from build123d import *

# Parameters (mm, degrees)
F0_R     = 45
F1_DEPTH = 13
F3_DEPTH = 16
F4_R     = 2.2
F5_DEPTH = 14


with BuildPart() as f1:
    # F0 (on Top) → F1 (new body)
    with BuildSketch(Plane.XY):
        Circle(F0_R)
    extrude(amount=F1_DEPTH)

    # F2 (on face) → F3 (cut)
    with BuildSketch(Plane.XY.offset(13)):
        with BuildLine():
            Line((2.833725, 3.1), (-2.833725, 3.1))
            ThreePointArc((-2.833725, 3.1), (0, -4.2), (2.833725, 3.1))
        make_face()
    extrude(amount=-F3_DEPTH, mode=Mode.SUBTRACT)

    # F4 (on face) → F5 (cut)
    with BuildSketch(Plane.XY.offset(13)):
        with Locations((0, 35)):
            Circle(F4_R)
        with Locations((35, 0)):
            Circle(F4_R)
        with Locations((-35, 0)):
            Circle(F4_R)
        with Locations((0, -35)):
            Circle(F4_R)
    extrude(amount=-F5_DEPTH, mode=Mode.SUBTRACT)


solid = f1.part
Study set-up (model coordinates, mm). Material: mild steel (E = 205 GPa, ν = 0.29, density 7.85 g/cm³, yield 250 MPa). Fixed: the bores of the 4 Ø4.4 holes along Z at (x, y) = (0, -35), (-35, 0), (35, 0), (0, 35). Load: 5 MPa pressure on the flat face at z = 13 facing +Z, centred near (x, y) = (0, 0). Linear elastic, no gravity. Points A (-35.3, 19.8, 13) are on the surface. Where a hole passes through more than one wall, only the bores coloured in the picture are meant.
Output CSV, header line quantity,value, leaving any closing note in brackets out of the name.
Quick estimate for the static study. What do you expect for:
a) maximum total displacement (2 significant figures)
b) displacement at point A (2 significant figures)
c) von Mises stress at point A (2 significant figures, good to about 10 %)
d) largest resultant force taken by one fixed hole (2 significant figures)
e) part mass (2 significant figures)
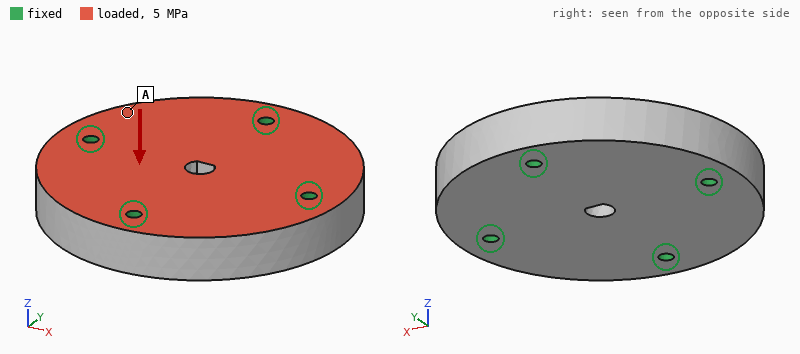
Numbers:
quantity,value
maximum total displacement,8.7 µm
displacement at point A,5.6 µm
von Mises stress at point A,15 MPa
largest resultant force taken by one fixed hole,7.8 kN
part mass,640 g
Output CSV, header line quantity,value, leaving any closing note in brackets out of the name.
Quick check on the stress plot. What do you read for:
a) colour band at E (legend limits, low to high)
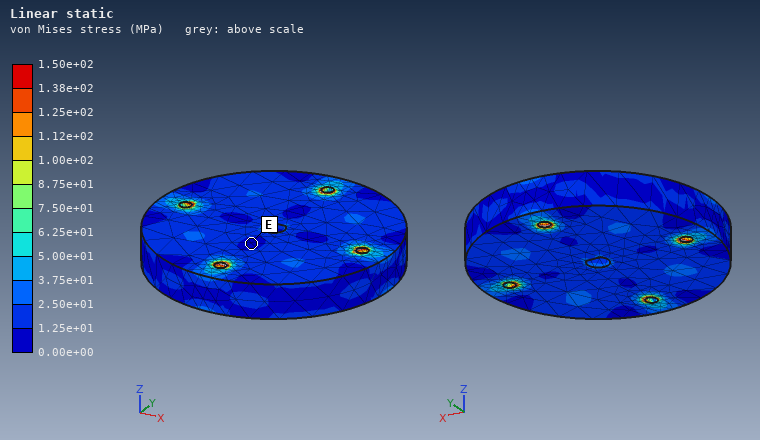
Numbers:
quantity,value
colour band at E,0.00e+00 to 1.25e+01 MPa
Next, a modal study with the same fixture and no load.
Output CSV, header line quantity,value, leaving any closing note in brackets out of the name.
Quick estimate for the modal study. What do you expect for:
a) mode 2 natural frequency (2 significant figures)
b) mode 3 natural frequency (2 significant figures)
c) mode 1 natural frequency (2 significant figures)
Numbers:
quantity,value
mode 2 natural frequency,14 kHz
mode 3 natural frequency,15 kHz
mode 1 natural frequency,14 kHz
